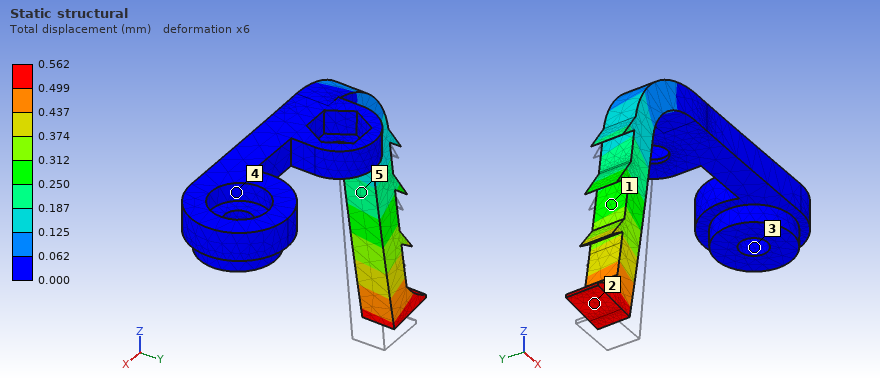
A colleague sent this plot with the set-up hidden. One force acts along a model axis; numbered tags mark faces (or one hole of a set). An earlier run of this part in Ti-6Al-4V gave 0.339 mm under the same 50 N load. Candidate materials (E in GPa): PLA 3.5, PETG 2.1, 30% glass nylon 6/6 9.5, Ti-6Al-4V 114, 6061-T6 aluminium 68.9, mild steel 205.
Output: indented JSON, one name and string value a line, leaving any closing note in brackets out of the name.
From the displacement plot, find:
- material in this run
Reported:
{
  "material in this run": "6061-T6 aluminium"
}
